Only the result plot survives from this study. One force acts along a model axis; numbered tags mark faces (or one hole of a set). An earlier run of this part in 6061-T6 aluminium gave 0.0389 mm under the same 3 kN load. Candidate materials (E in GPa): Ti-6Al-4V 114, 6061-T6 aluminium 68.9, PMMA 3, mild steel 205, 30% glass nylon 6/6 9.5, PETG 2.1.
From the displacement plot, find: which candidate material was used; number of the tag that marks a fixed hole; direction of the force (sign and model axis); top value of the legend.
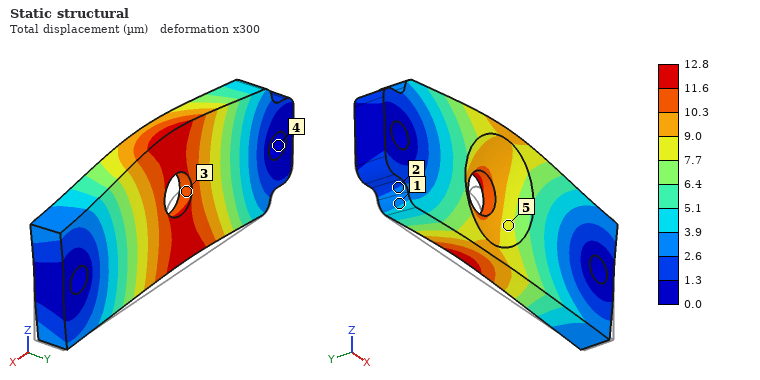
mild steel
4
+Z
12.8 µm
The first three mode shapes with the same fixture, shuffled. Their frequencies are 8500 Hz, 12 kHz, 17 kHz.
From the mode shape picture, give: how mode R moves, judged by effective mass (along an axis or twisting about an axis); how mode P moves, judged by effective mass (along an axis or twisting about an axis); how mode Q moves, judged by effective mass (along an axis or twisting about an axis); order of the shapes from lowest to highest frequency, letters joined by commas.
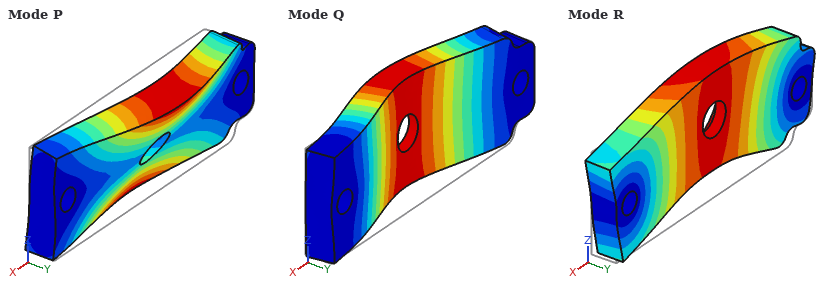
along Z
twisting about X
along Y
Q, P, R
